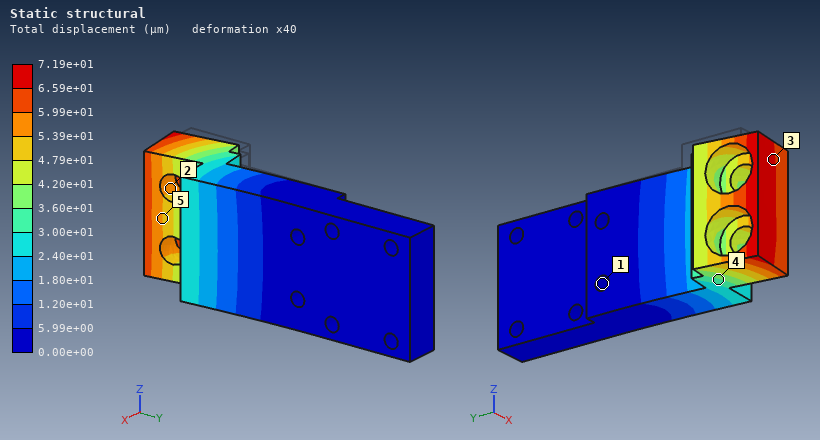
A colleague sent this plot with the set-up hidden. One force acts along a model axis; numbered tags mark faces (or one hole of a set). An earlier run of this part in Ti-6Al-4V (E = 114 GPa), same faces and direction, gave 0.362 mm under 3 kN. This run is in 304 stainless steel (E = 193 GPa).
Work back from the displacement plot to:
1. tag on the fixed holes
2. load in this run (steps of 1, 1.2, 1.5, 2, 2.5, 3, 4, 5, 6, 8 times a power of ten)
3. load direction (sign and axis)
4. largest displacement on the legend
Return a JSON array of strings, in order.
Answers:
["1", "1 kN", "+X", "7.19e+01 µm"]
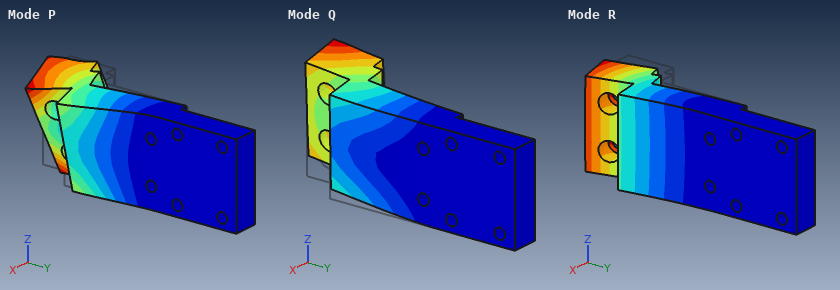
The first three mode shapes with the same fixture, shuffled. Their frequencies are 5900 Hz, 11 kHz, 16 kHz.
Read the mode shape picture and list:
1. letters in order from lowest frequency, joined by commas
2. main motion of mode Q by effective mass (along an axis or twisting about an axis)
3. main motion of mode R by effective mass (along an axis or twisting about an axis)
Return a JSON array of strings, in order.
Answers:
["R, Q, P", "along Z", "along X"]
